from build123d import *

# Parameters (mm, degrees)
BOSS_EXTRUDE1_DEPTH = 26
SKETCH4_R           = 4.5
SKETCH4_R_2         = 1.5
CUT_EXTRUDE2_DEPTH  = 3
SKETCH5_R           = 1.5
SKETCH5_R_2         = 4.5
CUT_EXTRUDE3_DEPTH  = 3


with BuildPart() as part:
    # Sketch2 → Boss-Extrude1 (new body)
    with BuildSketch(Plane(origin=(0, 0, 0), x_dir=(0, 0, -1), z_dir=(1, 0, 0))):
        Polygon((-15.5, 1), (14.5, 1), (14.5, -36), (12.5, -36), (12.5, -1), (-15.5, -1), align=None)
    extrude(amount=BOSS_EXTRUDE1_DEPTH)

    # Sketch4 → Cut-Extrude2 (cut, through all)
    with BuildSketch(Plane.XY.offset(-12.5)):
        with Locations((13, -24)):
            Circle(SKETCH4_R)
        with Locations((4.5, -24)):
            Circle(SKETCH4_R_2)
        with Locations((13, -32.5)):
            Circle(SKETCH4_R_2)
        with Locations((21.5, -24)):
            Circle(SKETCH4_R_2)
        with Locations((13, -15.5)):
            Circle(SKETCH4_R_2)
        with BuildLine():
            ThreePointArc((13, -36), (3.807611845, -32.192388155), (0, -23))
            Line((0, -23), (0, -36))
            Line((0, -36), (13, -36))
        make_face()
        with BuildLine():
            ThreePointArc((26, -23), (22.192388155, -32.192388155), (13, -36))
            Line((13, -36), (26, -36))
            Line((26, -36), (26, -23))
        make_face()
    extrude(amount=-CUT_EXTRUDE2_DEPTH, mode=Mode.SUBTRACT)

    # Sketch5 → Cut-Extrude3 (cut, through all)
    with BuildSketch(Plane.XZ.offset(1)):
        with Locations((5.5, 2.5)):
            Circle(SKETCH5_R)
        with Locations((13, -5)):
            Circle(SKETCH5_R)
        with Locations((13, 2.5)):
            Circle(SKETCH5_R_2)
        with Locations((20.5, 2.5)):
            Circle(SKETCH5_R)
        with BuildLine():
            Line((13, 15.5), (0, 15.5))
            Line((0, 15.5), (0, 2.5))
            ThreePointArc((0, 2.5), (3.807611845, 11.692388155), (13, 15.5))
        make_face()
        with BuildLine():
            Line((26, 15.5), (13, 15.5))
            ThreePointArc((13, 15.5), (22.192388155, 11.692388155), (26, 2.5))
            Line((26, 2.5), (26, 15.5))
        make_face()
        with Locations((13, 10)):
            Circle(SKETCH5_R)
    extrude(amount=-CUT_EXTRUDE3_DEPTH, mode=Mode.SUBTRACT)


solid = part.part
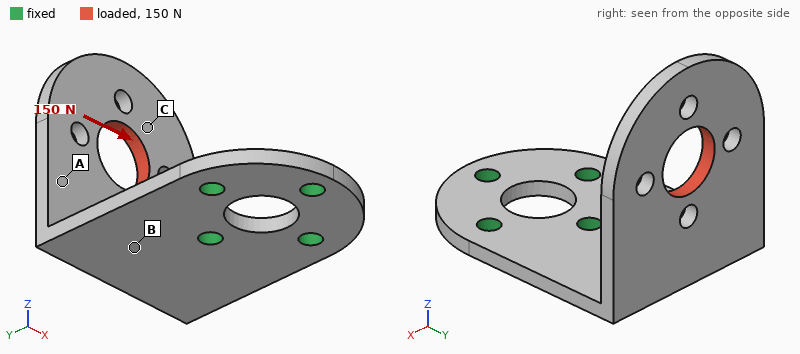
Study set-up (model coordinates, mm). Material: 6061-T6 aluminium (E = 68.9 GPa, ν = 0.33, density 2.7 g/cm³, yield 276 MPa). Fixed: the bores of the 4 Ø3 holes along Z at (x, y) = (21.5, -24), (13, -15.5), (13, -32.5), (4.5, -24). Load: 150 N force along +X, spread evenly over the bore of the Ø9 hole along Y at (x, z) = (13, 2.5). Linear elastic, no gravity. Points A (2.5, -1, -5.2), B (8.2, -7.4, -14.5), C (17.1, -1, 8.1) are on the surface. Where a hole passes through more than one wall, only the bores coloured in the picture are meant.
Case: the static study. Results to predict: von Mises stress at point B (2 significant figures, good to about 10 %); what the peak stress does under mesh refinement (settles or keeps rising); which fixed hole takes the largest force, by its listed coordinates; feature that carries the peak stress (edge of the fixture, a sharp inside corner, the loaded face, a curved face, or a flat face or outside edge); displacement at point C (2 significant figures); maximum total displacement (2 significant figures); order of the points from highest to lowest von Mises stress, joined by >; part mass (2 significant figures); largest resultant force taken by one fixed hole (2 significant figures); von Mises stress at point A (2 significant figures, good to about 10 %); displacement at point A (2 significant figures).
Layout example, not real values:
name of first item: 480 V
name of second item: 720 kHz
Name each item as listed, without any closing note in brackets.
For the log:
von Mises stress at point B: 79 MPa
what the peak stress does under mesh refinement: keeps rising
which fixed hole takes the largest force, by its listed coordinates: (13, -15.5)
feature that carries the peak stress: edge of the fixture
displacement at point C: 0.38 mm
maximum total displacement: 0.50 mm
order of the points from highest to lowest von Mises stress, joined by >: B > A > C
part mass: 7.4 g
largest resultant force taken by one fixed hole: 170 N
von Mises stress at point A: 31 MPa
displacement at point A: 0.23 mm
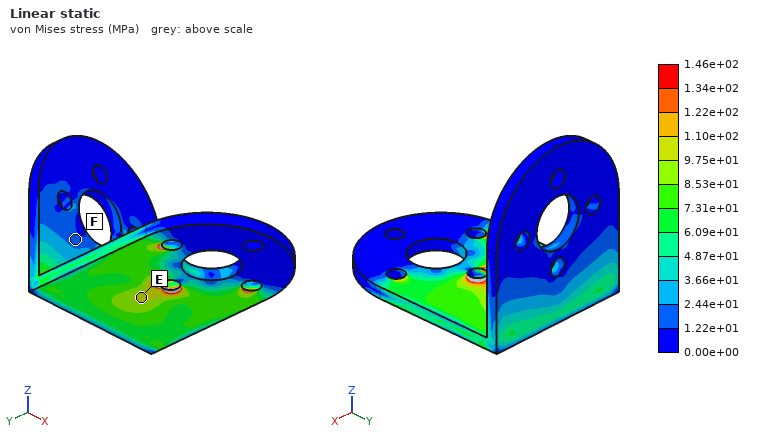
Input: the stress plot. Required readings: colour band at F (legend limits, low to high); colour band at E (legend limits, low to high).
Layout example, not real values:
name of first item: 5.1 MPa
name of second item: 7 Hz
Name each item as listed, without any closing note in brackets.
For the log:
colour band at F: 1.22e+01 to 2.44e+01 MPa
colour band at E: 9.75e+01 to 1.10e+02 MPa
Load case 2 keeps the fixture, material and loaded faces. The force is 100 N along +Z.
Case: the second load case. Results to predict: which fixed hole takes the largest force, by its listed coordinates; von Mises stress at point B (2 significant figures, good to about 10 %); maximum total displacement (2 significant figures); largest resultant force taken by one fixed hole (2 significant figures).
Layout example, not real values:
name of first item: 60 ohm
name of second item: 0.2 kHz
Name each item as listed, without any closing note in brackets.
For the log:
which fixed hole takes the largest force, by its listed coordinates: (13, -15.5)
von Mises stress at point B: 41 MPa
maximum total displacement: 0.32 mm
largest resultant force taken by one fixed hole: 160 N
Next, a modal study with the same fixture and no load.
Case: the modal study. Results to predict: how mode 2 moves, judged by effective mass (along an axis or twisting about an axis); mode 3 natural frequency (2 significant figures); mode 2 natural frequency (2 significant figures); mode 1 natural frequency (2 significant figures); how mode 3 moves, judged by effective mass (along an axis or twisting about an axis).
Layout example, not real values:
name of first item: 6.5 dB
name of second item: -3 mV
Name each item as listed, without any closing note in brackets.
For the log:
how mode 2 moves, judged by effective mass: along X
mode 3 natural frequency: 3600 Hz
mode 2 natural frequency: 1900 Hz
mode 1 natural frequency: 1300 Hz
how mode 3 moves, judged by effective mass: along Z
